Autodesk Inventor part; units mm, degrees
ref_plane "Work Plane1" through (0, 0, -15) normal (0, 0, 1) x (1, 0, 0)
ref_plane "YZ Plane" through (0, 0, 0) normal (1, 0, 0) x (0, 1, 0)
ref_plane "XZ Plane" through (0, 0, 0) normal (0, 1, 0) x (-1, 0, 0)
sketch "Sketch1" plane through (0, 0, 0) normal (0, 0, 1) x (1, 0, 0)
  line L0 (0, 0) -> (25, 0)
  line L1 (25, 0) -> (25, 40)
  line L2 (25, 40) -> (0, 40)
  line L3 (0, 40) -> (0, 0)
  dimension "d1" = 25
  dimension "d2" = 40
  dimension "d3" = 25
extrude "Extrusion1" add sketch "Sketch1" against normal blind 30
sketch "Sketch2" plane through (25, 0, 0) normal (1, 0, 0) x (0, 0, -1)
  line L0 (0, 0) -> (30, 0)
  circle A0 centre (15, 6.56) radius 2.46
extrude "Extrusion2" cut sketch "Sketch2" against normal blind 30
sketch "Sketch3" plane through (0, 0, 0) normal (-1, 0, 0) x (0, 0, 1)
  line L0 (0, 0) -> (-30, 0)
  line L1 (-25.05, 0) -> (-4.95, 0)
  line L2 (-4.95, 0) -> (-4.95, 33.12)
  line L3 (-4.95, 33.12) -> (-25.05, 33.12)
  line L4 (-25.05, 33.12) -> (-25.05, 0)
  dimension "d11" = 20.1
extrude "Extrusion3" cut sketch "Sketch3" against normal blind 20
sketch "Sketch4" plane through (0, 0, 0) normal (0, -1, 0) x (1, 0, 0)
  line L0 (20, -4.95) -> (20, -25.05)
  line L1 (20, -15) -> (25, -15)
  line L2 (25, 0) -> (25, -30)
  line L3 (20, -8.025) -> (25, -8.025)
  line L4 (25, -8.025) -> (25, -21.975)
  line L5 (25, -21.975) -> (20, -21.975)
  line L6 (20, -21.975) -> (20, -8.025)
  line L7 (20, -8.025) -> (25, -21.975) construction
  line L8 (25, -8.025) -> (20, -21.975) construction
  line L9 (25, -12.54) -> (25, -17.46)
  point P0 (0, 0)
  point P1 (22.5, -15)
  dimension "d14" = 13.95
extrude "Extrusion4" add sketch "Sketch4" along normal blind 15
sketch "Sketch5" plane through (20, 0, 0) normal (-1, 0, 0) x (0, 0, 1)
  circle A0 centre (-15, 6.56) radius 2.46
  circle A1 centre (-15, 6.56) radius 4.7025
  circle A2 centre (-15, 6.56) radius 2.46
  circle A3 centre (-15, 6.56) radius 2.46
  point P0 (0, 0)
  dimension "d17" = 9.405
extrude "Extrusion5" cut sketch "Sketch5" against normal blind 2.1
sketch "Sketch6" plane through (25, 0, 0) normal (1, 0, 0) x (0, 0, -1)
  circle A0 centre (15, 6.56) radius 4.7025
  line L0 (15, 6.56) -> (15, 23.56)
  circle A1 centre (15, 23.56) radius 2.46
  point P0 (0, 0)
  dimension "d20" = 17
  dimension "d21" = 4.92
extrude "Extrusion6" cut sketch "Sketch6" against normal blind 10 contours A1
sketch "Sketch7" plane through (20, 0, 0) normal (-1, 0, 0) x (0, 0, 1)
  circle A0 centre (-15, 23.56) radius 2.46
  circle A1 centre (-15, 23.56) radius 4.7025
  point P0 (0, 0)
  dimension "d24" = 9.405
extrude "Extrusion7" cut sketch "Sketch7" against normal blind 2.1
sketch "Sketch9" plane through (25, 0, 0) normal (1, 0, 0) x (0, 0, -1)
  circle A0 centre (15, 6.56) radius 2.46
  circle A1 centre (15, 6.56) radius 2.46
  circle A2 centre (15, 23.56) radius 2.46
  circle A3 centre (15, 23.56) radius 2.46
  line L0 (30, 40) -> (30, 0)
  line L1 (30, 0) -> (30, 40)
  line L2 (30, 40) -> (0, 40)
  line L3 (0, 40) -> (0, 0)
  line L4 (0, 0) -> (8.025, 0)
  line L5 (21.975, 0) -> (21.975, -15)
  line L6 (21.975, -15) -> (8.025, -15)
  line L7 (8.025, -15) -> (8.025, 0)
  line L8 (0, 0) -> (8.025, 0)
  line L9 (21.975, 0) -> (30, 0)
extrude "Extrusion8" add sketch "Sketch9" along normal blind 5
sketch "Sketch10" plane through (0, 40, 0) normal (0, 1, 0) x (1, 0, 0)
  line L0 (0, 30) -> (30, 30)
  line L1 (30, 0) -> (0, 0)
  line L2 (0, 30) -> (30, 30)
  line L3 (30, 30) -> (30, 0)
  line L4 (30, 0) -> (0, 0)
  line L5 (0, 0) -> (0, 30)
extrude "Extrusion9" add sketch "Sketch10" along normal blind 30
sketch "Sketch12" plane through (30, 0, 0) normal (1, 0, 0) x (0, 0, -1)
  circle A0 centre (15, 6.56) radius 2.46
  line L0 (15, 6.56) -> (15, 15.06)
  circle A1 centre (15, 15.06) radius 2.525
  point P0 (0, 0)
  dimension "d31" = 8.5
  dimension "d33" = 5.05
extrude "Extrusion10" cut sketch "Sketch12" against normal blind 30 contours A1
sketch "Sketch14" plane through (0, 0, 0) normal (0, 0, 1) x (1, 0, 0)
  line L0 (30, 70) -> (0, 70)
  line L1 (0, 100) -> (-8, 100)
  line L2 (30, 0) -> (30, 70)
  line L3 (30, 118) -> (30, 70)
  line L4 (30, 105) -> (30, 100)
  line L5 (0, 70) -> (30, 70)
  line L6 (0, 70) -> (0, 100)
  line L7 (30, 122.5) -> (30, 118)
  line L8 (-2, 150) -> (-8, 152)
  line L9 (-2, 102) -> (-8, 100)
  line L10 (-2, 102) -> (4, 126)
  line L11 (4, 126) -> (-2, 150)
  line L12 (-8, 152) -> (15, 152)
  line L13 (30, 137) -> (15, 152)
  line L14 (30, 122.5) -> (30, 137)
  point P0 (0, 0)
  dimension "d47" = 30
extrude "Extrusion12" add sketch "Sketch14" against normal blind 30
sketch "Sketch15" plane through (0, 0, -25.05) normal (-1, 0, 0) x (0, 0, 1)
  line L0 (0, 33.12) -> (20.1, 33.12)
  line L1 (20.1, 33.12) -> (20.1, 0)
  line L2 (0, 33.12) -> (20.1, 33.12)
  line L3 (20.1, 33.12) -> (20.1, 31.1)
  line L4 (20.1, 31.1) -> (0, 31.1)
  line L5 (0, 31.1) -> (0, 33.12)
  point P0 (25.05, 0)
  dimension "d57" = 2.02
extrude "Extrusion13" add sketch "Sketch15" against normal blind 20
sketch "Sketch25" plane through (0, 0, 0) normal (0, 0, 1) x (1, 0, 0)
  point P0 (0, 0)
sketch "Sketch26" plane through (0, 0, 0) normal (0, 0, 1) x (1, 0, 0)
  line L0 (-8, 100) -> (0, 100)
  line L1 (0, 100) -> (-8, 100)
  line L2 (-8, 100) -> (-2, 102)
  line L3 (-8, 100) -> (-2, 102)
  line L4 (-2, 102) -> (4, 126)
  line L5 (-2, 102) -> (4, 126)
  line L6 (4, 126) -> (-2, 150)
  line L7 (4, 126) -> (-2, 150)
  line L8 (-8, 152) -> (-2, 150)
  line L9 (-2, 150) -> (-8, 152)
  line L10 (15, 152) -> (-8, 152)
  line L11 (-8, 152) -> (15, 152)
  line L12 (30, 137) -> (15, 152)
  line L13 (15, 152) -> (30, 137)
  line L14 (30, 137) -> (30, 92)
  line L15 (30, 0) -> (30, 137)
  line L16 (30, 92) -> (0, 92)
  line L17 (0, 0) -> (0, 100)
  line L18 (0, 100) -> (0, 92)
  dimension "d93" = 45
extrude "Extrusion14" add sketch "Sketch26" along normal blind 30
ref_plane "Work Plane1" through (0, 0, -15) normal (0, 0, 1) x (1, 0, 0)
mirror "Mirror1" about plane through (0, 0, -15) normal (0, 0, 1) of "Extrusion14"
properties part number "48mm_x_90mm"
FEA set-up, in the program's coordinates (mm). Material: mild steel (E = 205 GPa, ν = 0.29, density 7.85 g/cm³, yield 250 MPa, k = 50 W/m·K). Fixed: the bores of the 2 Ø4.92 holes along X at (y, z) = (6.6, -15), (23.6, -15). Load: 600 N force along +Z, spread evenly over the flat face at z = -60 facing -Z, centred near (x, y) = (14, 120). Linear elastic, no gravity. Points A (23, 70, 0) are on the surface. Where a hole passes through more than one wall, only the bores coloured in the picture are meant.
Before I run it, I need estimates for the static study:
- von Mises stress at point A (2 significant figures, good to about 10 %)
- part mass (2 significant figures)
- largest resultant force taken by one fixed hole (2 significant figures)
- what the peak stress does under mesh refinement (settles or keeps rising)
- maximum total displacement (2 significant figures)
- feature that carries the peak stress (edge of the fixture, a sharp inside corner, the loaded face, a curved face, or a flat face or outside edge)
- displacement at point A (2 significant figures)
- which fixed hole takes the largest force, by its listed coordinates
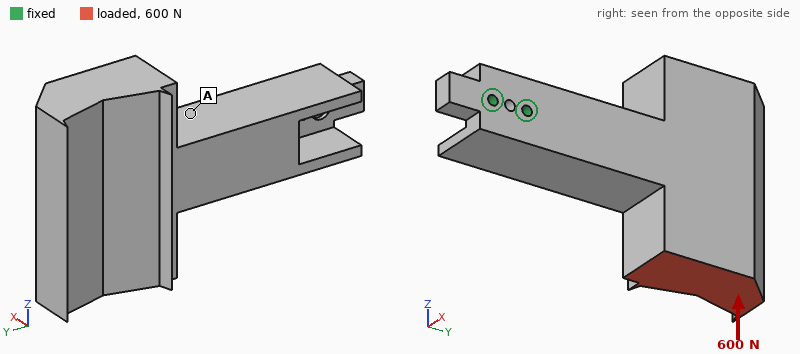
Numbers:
6.8 MPa
1.7 kg
3.1 kN
keeps rising
58 µm
edge of the fixture
17 µm
(23.6, -15)
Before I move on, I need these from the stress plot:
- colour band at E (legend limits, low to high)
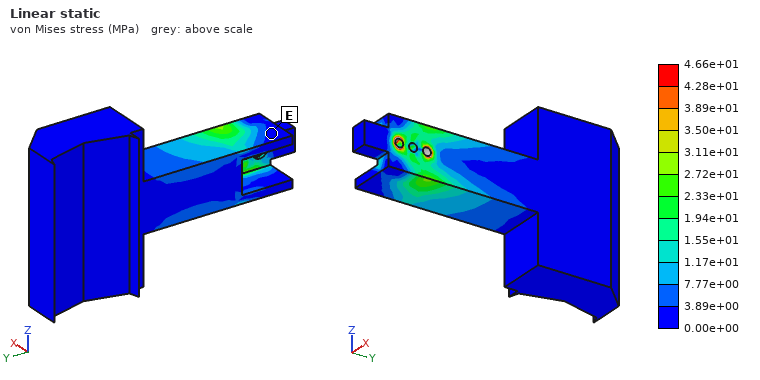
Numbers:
0.00e+00 to 3.89e+00 MPa
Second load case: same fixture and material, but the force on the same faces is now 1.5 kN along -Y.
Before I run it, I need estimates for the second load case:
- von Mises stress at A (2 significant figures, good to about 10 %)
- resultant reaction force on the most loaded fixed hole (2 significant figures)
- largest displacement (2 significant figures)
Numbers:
14 MPa
3.1 kN
85 µm
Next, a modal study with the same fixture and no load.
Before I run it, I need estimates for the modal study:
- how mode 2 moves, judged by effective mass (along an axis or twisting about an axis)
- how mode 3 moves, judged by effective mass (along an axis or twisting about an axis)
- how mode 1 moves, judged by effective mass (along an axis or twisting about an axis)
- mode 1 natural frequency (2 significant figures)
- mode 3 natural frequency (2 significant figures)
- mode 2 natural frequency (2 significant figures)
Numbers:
along Z
twisting about Y
along X
470 Hz
1100 Hz
530 Hz
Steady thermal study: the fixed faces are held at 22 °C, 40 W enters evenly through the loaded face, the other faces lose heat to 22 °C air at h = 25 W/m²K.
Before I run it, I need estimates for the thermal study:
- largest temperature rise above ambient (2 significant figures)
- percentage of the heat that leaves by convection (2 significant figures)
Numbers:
59 K
62 %
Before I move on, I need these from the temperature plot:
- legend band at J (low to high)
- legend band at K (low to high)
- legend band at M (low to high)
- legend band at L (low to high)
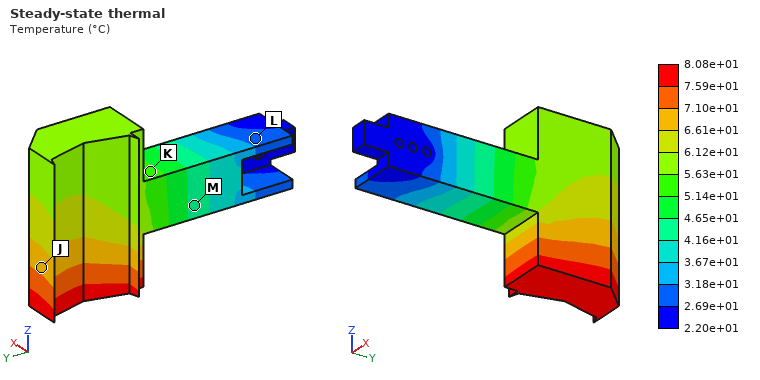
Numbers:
6.61e+01 to 7.10e+01 °C
5.14e+01 to 5.63e+01 °C
4.16e+01 to 4.65e+01 °C
2.69e+01 to 3.18e+01 °C
